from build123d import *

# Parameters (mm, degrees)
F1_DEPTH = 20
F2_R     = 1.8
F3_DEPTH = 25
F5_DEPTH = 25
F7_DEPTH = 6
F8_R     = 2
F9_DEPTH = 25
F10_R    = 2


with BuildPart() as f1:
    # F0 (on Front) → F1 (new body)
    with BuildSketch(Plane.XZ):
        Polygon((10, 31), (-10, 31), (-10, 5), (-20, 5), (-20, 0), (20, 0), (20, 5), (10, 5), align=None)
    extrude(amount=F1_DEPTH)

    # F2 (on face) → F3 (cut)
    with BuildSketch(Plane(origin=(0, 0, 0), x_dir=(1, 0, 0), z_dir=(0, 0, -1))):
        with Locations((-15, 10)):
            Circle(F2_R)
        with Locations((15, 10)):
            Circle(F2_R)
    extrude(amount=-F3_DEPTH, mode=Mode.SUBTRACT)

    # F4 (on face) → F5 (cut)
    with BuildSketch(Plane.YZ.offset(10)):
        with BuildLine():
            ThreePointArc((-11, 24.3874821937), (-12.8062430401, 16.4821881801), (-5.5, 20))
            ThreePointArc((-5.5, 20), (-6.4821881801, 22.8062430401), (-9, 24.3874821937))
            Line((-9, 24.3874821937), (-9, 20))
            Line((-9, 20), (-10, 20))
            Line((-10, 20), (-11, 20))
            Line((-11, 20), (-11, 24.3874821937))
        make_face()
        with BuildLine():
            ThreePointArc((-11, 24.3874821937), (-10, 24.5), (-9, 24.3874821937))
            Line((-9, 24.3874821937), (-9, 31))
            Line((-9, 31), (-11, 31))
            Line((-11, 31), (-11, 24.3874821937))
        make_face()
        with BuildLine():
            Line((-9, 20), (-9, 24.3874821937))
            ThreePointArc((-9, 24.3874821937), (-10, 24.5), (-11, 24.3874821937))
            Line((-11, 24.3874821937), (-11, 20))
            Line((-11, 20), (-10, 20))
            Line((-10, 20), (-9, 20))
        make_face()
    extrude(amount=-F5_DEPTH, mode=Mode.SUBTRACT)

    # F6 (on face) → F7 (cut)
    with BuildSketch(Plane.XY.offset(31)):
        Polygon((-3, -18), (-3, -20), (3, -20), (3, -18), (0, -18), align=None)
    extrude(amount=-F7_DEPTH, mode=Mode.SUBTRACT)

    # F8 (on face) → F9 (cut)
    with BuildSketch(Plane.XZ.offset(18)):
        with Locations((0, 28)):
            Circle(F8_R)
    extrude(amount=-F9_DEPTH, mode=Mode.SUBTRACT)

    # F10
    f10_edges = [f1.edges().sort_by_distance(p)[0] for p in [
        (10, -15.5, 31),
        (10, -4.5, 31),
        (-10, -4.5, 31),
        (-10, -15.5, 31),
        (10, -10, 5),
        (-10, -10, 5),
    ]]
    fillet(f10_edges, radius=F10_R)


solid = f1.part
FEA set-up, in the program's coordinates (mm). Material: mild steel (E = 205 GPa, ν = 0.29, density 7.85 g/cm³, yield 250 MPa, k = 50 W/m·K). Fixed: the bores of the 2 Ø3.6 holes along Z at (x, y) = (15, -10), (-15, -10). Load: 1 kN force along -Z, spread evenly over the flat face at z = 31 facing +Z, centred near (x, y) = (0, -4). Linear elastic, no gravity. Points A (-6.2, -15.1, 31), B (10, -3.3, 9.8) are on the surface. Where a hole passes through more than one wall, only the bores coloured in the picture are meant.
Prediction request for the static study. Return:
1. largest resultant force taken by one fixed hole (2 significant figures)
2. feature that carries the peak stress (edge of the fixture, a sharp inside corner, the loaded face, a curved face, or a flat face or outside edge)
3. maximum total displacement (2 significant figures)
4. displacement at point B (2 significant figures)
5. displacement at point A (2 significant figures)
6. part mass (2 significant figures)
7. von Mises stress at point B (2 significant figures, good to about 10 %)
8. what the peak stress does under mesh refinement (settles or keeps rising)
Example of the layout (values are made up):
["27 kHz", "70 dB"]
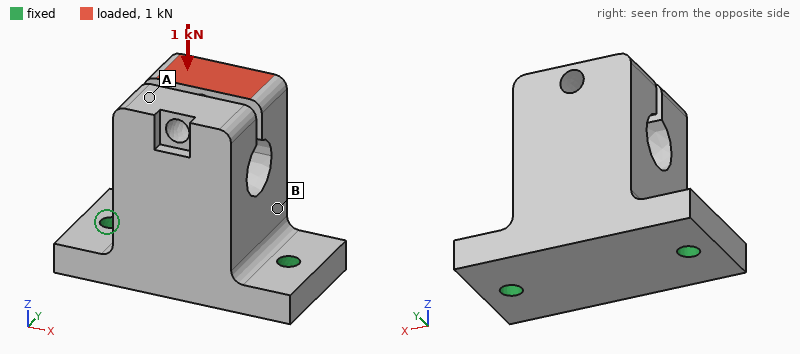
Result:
["540 N", "edge of the fixture", "8.6 µm", "3.9 µm", "8.4 µm", "98 g", "11 MPa", "keeps rising"]
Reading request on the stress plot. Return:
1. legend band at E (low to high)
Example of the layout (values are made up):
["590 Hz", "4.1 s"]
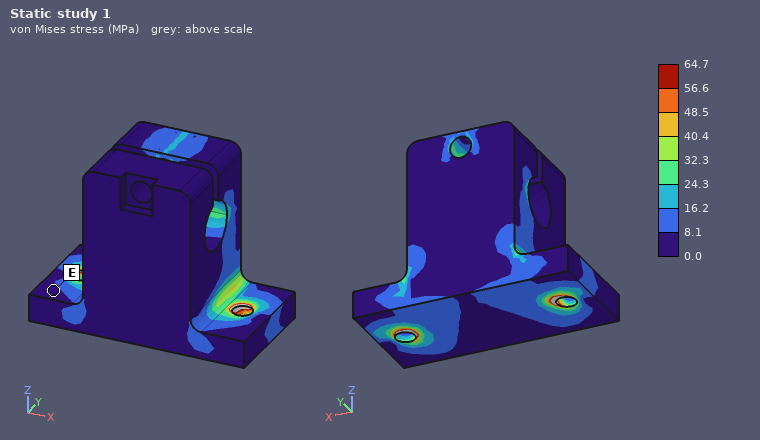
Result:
["0.0 to 8.1 MPa"]
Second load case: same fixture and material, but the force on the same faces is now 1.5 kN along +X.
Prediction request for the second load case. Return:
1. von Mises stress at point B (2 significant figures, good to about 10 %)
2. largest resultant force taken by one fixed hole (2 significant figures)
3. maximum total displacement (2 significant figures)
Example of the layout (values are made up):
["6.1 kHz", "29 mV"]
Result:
["52 MPa", "1.8 kN", "22 µm"]
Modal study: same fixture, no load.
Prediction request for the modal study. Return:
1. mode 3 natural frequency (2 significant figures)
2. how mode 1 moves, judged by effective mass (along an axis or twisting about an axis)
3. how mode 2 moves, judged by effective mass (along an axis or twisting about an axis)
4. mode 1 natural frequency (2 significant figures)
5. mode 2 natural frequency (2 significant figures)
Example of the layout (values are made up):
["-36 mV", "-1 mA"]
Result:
["13 kHz", "along Y", "along X", "4400 Hz", "11 kHz"]
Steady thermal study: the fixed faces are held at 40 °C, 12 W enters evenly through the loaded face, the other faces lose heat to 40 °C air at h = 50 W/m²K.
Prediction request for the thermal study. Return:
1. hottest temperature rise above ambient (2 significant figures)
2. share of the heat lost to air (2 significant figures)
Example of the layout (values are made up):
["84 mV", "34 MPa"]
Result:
["49 K", "25 %"]
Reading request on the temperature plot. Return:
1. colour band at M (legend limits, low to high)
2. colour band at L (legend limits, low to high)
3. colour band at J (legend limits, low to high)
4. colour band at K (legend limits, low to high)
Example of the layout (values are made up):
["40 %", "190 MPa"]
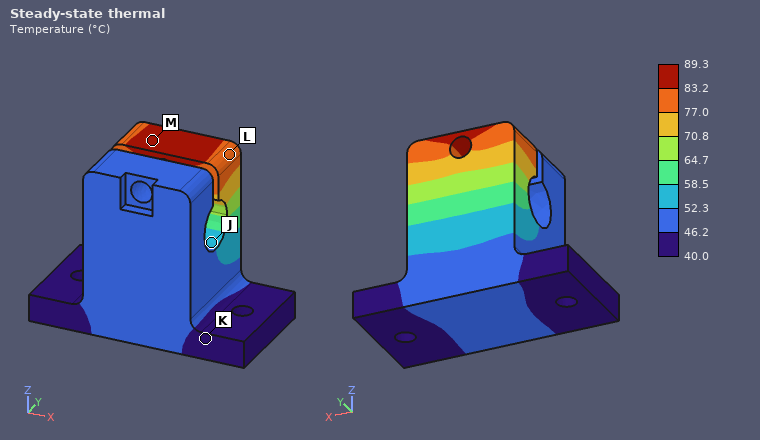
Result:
["83.2 to 89.3 °C", "77.0 to 83.2 °C", "52.3 to 58.5 °C", "40.0 to 46.2 °C"]
